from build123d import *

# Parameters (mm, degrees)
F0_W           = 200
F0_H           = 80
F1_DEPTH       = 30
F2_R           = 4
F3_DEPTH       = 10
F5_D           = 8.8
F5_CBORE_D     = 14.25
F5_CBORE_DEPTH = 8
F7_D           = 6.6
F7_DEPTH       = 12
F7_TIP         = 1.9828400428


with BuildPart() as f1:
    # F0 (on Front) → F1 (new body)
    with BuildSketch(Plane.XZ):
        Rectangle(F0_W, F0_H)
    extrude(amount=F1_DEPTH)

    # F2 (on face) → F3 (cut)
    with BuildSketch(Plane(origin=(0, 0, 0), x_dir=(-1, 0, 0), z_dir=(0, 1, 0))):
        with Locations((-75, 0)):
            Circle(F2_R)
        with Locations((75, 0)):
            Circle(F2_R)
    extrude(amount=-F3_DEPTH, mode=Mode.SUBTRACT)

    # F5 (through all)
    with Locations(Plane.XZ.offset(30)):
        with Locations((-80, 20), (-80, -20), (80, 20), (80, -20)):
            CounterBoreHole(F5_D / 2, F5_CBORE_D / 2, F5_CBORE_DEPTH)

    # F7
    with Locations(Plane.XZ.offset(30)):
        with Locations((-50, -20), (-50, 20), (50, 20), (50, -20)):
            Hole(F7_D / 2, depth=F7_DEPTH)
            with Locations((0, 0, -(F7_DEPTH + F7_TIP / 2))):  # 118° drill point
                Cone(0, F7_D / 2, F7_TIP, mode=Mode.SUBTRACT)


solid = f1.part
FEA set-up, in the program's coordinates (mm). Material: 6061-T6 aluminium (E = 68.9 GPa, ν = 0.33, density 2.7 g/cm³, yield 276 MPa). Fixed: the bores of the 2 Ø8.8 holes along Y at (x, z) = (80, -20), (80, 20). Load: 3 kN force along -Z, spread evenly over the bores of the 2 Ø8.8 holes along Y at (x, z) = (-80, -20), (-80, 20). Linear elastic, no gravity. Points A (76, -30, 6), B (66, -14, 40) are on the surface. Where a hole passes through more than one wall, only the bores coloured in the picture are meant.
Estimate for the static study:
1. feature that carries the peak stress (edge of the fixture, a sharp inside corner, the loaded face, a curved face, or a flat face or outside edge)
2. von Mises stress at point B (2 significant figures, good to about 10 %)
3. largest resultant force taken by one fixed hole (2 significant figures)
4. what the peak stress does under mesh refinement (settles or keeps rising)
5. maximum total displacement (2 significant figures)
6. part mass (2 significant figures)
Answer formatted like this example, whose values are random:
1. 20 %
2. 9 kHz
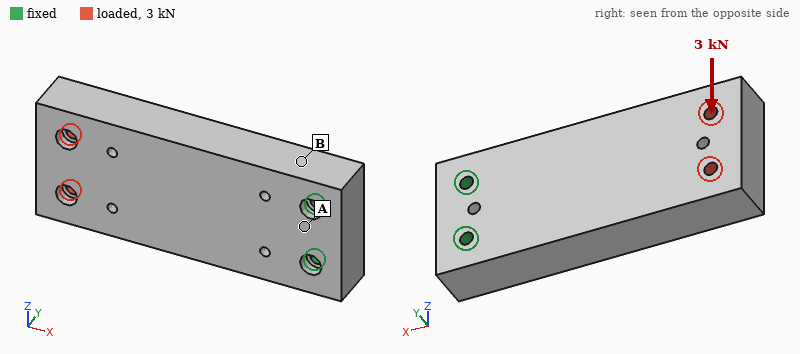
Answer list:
1. edge of the fixture
2. 10 MPa
3. 11 kN
4. keeps rising
5. 92 µm
6. 1.3 kg
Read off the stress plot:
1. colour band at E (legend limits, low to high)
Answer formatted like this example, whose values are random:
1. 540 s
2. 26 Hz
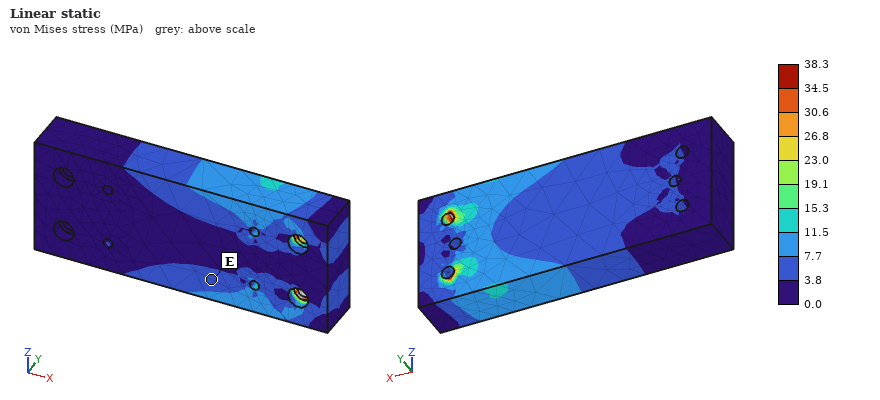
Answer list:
1. 3.8 to 7.7 MPa
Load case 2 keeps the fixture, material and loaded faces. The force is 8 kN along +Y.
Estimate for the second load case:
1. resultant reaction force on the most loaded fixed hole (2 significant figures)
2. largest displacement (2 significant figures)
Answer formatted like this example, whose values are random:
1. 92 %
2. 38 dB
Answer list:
1. 4.4 kN
2. 1.4 mm
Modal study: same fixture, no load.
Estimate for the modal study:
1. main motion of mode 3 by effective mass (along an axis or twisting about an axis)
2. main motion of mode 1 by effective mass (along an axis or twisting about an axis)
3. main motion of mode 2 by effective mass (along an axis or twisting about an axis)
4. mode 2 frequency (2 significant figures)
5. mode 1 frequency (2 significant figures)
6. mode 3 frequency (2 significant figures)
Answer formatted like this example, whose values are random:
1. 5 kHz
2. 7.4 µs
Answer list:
1. twisting about X
2. along Y
3. along Z
4. 1500 Hz
5. 650 Hz
6. 2700 Hz
